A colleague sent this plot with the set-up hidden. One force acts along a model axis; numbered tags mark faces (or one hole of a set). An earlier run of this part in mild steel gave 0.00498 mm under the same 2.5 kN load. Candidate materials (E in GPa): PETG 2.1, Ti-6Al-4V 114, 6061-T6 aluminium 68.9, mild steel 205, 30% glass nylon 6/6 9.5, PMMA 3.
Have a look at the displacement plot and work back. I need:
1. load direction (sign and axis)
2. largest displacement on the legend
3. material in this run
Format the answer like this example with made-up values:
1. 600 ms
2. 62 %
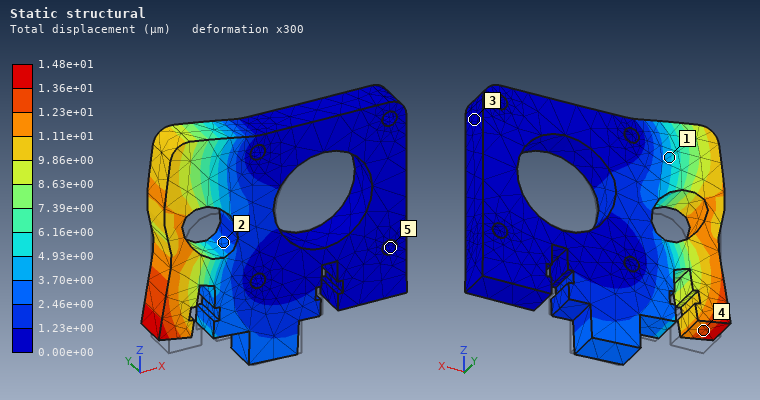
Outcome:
1. +Z
2. 1.48e+01 µm
3. 6061-T6 aluminium
